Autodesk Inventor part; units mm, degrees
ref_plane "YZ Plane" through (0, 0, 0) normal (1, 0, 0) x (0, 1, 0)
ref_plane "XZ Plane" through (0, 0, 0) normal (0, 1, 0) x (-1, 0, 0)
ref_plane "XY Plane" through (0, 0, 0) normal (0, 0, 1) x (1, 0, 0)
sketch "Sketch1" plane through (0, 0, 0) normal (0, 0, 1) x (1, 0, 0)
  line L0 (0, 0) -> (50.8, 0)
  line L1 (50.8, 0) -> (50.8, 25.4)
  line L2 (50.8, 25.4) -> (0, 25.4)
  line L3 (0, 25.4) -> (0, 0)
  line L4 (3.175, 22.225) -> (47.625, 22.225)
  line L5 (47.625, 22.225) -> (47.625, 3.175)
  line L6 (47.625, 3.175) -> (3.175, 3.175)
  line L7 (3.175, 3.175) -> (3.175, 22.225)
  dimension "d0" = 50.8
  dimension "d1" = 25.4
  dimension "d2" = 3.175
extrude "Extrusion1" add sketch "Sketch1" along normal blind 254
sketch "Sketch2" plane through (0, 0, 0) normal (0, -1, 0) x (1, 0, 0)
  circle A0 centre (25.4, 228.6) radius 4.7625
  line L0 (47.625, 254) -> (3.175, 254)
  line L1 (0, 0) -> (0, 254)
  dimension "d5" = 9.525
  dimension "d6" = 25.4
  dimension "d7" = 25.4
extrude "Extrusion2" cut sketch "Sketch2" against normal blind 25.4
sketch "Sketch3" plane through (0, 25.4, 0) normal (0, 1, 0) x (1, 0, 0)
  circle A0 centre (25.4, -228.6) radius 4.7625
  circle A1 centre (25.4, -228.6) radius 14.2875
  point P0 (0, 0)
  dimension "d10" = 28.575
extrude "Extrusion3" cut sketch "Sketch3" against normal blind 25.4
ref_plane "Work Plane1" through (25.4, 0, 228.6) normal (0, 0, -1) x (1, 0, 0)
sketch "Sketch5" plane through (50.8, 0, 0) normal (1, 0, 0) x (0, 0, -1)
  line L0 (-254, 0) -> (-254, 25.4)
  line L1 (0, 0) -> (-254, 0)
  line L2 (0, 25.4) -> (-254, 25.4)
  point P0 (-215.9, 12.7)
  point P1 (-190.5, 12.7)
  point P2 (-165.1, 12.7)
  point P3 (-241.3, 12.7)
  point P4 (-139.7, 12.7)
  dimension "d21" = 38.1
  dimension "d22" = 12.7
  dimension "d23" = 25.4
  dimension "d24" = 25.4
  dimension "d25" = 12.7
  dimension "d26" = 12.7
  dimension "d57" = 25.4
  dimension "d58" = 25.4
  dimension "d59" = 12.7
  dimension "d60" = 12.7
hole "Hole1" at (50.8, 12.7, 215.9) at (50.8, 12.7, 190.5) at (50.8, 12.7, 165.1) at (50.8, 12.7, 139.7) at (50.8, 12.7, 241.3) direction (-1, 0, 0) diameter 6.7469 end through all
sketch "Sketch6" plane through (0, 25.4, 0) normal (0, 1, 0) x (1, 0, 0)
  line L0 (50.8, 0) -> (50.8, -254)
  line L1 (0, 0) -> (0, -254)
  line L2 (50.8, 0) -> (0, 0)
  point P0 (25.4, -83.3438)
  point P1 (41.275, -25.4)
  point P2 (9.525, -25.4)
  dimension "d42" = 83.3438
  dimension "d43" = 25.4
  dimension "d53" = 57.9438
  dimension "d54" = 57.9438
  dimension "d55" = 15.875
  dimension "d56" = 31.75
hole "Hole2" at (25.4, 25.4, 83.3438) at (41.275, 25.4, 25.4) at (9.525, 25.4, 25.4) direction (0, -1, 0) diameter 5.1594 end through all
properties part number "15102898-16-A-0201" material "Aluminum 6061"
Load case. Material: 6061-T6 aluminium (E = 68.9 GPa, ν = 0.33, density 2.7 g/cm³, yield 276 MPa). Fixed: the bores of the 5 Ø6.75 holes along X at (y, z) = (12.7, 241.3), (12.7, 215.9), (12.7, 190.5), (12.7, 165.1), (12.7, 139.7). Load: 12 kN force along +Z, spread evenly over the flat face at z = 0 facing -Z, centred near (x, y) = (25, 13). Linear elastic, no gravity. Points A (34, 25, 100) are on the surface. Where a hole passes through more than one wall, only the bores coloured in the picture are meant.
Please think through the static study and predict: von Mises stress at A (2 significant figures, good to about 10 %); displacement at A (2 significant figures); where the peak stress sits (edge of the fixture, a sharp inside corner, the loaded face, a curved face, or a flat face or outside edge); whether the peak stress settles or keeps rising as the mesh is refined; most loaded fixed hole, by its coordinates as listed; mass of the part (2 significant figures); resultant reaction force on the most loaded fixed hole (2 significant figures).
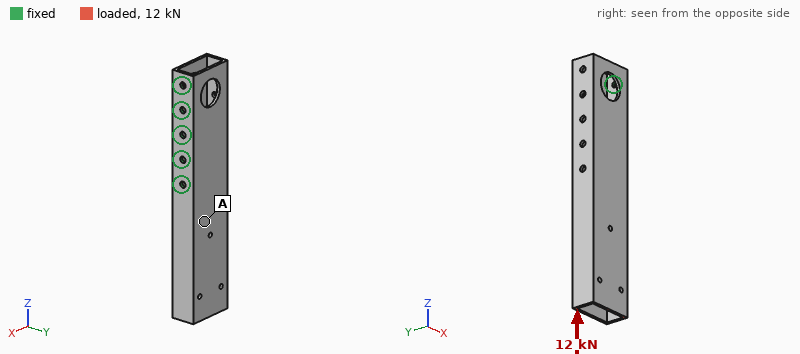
22 MPa
0.13 mm
edge of the fixture
keeps rising
(12.7, 139.7)
290 g
5.2 kN
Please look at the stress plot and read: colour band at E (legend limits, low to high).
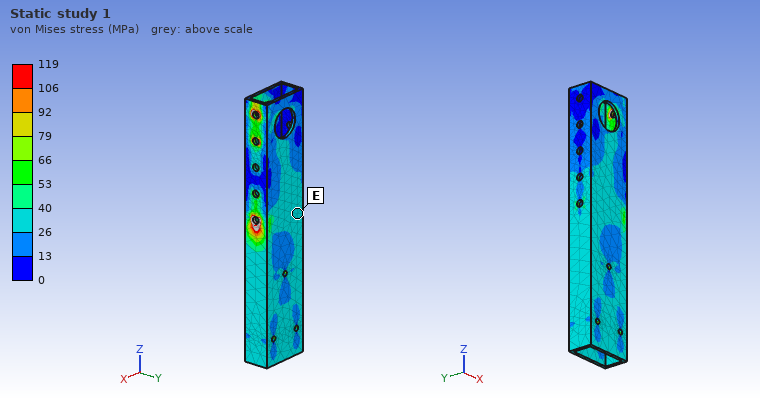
26 to 40 MPa
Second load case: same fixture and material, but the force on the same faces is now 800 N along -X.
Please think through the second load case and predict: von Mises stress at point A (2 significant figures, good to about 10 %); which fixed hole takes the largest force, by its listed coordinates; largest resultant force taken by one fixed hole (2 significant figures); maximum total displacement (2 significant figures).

8.0 MPa
(12.7, 139.7)
2.3 kN
0.26 mm
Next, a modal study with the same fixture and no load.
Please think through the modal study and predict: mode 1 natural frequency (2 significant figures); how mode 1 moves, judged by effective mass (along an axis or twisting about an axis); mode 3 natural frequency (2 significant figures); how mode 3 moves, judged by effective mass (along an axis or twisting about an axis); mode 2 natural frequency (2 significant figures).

660 Hz
along Y
1100 Hz
along X
1000 Hz
